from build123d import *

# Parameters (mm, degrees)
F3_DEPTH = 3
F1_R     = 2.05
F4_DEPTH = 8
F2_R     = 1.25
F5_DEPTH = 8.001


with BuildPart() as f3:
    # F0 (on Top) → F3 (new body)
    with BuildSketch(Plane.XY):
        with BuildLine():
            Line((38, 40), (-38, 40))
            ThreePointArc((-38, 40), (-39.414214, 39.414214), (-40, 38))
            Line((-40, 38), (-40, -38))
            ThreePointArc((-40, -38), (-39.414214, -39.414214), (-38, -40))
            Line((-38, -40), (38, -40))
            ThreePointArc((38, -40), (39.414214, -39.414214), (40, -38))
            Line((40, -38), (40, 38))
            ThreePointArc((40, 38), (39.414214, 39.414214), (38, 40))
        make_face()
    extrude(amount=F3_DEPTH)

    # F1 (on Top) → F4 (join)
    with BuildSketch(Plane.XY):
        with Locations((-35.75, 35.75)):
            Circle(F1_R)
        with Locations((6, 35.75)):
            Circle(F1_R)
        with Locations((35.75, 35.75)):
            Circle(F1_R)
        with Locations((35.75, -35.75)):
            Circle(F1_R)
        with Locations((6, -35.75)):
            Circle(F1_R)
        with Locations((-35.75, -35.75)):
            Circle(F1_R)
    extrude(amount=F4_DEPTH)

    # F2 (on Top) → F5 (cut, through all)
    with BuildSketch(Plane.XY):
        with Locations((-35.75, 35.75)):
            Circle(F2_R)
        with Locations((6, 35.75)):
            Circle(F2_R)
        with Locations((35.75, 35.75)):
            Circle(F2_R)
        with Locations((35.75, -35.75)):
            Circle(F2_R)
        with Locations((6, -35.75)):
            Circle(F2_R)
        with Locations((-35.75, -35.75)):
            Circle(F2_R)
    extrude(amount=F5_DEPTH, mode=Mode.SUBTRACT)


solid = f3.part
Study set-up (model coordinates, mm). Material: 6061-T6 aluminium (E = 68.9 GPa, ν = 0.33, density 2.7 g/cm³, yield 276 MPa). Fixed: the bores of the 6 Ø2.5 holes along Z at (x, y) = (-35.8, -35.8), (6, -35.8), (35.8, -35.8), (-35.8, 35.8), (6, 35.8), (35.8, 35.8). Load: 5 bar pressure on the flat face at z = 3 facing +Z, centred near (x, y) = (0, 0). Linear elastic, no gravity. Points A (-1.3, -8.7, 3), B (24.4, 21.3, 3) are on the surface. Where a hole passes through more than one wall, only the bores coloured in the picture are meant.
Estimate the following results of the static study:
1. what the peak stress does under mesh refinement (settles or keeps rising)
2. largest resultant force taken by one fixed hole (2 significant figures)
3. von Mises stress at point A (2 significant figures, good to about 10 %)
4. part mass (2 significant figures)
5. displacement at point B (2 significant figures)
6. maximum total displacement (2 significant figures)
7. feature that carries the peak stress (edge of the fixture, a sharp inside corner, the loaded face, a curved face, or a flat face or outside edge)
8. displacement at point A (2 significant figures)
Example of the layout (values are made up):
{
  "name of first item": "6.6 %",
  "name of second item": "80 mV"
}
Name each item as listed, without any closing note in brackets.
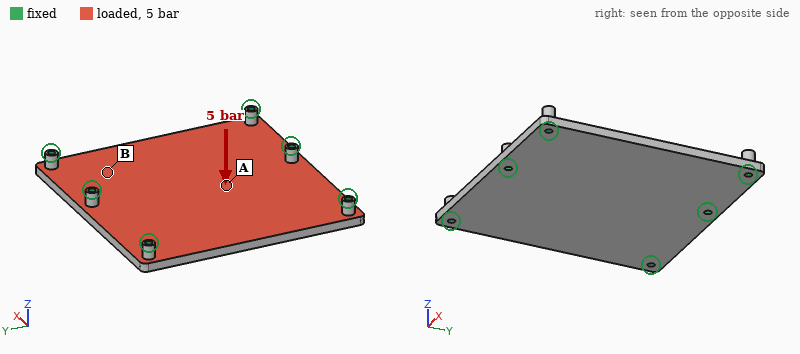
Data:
{
  "what the peak stress does under mesh refinement": "keeps rising",
  "largest resultant force taken by one fixed hole": "740 N",
  "von Mises stress at point A": "66 MPa",
  "part mass": "52 g",
  "displacement at point B": "0.14 mm",
  "maximum total displacement": "0.32 mm",
  "feature that carries the peak stress": "edge of the fixture",
  "displacement at point A": "0.28 mm"
}
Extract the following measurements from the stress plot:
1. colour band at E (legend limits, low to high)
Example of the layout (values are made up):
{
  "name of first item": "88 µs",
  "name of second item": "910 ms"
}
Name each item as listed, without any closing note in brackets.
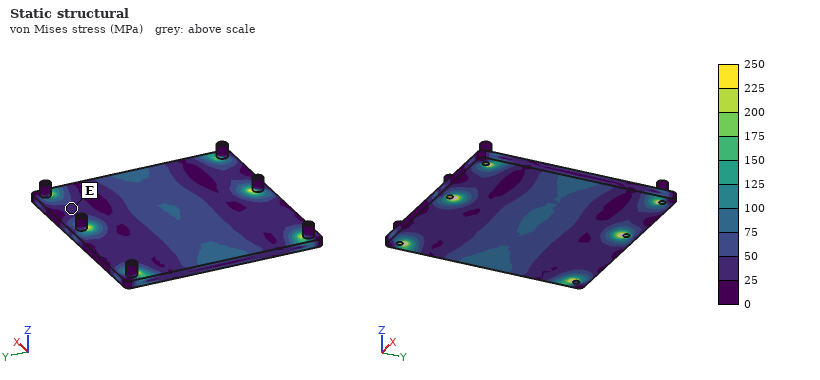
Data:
{
  "colour band at E": "25 to 50 MPa"
}
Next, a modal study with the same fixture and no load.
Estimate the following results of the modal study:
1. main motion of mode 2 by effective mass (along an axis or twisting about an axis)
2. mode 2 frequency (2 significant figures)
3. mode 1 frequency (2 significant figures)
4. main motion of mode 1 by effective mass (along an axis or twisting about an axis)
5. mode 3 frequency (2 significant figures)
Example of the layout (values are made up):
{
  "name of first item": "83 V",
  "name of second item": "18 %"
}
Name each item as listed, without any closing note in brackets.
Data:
{
  "main motion of mode 2 by effective mass": "twisting about Y",
  "mode 2 frequency": "3300 Hz",
  "mode 1 frequency": "2600 Hz",
  "main motion of mode 1 by effective mass": "along Z",
  "mode 3 frequency": "5300 Hz"
}
